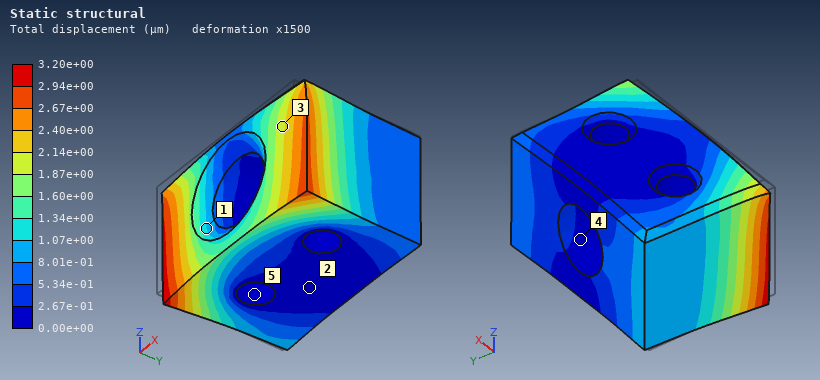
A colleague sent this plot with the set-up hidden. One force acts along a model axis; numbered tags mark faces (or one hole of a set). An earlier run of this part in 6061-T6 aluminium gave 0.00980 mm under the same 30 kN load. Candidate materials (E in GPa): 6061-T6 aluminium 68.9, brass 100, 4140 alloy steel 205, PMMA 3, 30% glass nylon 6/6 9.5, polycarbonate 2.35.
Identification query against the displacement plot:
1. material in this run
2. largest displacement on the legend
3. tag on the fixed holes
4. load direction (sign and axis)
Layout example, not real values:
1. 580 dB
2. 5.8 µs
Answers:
1. 4140 alloy steel
2. 3.20e+00 µm
3. 5
4. +Y
